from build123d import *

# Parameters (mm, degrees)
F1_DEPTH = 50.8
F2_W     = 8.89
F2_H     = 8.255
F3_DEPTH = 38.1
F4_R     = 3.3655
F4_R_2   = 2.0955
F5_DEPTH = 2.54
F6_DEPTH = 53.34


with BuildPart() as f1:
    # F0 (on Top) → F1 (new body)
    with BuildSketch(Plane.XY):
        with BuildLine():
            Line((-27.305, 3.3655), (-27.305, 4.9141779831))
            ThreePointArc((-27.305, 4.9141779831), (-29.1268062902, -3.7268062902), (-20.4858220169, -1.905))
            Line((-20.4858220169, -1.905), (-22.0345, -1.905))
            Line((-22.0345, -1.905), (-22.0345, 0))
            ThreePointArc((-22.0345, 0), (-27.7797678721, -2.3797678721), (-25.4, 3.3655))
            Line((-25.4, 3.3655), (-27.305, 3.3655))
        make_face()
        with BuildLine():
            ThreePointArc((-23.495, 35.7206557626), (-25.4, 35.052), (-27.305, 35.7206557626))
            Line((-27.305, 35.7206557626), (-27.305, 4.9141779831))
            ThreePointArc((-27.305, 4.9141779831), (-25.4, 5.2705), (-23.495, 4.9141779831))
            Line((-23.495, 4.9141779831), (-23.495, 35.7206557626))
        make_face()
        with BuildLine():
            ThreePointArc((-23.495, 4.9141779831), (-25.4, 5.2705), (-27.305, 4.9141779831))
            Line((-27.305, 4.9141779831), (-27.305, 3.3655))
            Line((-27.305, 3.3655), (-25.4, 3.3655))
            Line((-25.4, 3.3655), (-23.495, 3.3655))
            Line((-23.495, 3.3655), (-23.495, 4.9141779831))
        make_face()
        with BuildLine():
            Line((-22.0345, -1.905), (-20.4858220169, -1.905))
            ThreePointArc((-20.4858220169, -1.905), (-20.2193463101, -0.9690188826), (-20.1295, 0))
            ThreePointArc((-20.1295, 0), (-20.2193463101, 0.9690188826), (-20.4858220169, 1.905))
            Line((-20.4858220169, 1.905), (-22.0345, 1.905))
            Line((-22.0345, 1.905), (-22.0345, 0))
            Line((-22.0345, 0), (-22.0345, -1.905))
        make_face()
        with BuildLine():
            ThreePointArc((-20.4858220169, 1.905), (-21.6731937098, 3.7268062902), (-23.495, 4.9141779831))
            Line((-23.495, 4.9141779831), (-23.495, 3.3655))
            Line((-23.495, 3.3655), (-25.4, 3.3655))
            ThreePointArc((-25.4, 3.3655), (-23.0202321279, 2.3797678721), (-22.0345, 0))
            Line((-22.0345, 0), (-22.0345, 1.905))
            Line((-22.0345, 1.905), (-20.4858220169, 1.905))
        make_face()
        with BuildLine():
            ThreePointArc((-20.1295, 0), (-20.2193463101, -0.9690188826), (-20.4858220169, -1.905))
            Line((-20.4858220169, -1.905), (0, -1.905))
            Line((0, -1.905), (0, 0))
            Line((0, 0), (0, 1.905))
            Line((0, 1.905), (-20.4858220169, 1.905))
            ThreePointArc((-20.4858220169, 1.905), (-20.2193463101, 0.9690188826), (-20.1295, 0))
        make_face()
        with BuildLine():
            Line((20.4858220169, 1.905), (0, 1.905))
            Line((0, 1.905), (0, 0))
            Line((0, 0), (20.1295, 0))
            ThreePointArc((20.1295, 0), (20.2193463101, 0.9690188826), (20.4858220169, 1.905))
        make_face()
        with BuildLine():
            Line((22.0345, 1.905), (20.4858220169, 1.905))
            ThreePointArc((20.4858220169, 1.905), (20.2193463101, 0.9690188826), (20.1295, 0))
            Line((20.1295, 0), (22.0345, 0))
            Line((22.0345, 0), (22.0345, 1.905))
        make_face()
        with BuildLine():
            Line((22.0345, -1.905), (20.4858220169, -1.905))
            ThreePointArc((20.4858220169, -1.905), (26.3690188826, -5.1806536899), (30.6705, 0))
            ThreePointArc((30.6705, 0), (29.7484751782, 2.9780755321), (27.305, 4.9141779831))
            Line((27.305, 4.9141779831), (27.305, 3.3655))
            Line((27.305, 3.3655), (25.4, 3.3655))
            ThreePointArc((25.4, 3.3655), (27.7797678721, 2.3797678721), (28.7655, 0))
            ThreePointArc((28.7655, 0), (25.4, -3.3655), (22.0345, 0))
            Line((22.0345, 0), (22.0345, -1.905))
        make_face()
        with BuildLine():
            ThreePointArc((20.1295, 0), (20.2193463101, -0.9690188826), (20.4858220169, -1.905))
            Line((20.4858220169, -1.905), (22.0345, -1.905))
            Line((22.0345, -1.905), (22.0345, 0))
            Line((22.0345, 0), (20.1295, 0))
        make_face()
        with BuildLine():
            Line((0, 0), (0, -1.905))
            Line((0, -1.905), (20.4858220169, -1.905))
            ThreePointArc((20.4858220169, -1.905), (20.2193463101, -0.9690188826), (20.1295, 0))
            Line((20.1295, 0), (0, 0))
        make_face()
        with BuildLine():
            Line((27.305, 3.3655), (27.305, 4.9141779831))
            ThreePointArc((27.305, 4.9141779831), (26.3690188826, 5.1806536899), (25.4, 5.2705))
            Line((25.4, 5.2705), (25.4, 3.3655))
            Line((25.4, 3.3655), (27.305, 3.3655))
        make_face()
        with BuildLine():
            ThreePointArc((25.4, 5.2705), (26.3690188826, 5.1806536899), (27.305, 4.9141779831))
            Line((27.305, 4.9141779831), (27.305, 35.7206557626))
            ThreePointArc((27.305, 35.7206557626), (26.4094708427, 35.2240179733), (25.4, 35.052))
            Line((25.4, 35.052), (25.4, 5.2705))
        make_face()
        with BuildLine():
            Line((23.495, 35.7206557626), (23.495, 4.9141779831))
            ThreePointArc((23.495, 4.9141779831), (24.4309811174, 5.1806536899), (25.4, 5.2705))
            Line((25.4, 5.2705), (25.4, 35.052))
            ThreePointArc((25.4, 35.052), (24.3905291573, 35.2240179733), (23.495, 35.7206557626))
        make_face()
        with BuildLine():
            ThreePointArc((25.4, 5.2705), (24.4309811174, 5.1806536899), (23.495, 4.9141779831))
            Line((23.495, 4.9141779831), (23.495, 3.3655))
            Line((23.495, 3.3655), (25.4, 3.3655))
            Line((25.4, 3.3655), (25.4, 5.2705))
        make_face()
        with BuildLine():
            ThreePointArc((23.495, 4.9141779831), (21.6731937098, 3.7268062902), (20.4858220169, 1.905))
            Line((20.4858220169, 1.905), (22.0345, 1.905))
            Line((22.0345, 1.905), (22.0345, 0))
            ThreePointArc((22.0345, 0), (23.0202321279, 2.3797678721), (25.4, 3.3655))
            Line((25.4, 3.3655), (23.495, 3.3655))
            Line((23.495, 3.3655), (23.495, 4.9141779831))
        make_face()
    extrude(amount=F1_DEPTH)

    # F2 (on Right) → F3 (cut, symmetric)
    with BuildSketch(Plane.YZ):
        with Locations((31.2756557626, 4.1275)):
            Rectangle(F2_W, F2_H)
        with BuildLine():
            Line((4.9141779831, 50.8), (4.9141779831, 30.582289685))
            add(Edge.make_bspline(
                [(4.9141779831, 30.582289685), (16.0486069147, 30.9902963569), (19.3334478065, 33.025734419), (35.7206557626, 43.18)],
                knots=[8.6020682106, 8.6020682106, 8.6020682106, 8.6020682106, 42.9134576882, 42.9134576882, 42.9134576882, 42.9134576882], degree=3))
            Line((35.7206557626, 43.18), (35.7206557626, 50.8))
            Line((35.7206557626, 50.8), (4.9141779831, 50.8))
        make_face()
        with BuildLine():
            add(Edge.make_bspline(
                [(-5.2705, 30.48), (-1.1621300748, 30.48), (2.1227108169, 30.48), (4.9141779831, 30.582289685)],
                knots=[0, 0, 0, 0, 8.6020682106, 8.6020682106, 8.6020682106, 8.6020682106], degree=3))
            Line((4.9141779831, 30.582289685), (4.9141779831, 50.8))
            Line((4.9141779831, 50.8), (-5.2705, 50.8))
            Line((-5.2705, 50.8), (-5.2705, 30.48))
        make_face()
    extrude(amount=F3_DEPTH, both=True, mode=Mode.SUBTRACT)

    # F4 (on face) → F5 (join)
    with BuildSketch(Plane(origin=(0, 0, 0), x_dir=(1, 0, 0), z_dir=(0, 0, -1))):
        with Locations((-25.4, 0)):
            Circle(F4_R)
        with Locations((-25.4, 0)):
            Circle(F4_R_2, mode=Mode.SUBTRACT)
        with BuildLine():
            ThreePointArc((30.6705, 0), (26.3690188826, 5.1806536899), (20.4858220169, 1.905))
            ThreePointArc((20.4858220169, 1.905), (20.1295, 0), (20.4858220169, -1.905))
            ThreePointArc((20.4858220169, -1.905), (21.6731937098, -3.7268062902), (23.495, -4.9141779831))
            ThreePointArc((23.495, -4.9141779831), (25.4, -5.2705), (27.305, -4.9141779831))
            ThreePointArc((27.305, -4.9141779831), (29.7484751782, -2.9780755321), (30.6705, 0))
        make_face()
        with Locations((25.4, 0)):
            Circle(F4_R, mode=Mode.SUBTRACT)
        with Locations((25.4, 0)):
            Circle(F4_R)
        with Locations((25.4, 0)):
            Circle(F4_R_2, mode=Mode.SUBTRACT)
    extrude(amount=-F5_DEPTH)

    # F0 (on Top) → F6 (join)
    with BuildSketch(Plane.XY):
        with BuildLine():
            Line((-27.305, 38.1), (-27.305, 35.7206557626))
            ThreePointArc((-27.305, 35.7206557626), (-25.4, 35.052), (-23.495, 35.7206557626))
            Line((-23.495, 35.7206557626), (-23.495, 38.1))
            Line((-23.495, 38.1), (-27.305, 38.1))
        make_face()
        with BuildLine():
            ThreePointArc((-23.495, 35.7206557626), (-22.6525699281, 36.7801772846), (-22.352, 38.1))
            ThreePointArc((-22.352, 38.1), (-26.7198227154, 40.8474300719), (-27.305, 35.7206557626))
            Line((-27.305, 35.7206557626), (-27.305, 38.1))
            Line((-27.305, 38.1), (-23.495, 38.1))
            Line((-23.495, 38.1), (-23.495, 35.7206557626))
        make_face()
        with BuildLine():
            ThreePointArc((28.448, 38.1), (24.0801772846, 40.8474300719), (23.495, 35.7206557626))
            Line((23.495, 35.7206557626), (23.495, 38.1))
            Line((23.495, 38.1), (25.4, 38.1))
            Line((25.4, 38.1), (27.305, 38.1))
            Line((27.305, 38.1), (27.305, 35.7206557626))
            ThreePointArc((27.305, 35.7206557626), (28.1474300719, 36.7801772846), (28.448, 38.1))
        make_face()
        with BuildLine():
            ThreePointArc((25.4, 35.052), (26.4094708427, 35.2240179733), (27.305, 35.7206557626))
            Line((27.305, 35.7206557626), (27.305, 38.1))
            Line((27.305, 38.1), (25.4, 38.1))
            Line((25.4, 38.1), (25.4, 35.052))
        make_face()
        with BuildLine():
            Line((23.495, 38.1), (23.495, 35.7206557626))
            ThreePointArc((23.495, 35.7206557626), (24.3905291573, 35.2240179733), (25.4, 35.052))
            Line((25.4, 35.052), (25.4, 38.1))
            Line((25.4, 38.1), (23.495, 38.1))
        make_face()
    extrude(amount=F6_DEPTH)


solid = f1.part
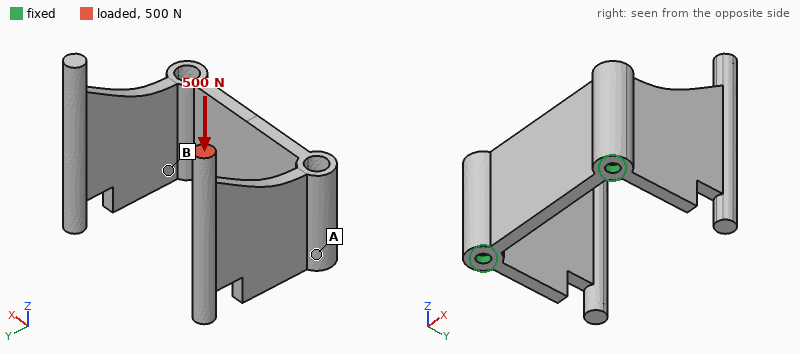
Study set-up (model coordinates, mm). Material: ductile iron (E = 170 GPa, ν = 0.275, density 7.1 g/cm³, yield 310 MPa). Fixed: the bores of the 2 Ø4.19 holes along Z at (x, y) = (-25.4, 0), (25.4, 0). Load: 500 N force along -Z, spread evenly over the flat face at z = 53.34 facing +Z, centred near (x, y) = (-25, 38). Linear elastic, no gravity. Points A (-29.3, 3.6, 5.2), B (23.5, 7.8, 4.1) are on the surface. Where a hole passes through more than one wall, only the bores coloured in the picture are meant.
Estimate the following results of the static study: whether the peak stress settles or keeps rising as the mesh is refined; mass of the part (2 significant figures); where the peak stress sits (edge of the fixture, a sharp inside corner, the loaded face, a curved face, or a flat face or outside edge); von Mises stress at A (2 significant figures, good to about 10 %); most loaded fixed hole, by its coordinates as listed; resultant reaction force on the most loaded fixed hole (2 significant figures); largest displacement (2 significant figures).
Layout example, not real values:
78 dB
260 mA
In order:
keeps rising
130 g
edge of the fixture
72 MPa
(-25.4, 0)
510 N
0.25 mm
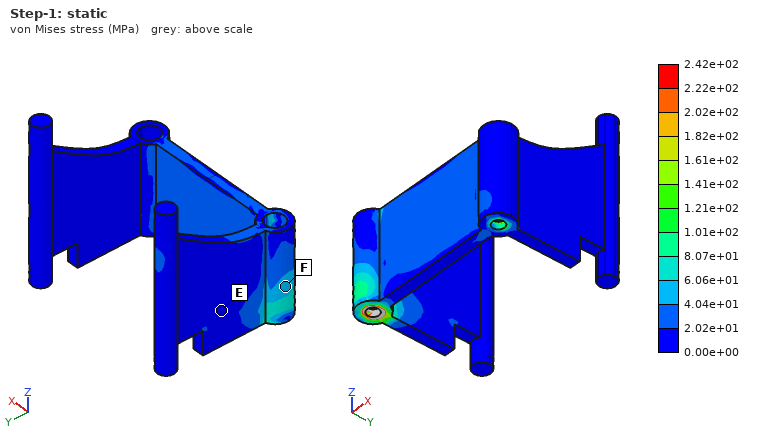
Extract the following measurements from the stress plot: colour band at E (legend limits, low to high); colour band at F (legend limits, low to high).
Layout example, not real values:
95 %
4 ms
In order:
0.00e+00 to 2.02e+01 MPa
4.04e+01 to 6.06e+01 MPa
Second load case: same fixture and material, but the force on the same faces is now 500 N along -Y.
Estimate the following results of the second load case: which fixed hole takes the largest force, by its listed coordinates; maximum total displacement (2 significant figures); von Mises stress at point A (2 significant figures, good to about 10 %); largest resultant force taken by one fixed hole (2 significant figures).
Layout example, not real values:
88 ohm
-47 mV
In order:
(-25.4, 0)
0.38 mm
93 MPa
440 N
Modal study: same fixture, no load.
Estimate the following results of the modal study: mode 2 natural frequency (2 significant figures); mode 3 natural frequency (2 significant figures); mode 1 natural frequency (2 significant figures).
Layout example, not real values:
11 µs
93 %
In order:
1200 Hz
1400 Hz
1200 Hz
